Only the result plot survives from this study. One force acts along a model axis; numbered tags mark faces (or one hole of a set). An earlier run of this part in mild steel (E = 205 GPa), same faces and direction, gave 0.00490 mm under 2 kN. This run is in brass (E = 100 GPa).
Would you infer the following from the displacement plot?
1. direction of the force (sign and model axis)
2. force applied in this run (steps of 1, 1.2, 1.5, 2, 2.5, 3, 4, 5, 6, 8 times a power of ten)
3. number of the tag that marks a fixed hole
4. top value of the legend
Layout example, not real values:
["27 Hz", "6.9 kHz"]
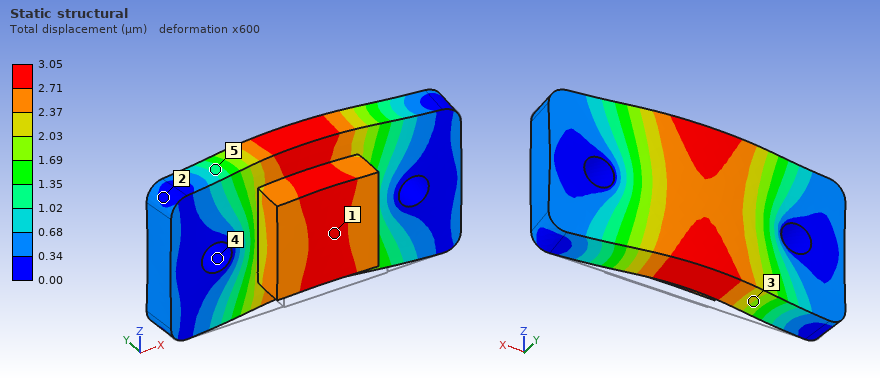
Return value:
["+Y", "600 N", "4", "3.05 µm"]
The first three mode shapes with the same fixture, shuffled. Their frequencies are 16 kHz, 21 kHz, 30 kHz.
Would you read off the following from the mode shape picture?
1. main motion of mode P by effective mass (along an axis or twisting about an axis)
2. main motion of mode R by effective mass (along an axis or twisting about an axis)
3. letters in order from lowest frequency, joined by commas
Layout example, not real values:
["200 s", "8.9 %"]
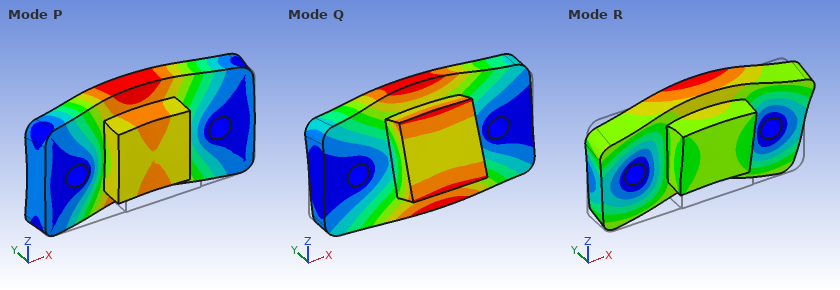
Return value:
["along Y", "along Z", "Q, P, R"]
